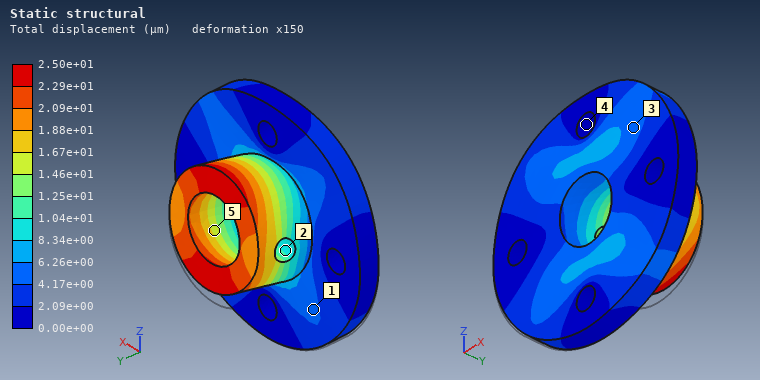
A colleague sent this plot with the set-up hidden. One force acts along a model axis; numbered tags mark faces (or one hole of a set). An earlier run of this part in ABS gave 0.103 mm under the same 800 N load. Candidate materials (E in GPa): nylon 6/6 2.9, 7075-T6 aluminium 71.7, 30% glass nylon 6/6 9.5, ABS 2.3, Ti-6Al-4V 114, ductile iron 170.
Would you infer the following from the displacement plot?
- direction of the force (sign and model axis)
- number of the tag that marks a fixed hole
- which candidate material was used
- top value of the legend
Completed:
+Z
4
30% glass nylon 6/6
2.50e+01 µm
